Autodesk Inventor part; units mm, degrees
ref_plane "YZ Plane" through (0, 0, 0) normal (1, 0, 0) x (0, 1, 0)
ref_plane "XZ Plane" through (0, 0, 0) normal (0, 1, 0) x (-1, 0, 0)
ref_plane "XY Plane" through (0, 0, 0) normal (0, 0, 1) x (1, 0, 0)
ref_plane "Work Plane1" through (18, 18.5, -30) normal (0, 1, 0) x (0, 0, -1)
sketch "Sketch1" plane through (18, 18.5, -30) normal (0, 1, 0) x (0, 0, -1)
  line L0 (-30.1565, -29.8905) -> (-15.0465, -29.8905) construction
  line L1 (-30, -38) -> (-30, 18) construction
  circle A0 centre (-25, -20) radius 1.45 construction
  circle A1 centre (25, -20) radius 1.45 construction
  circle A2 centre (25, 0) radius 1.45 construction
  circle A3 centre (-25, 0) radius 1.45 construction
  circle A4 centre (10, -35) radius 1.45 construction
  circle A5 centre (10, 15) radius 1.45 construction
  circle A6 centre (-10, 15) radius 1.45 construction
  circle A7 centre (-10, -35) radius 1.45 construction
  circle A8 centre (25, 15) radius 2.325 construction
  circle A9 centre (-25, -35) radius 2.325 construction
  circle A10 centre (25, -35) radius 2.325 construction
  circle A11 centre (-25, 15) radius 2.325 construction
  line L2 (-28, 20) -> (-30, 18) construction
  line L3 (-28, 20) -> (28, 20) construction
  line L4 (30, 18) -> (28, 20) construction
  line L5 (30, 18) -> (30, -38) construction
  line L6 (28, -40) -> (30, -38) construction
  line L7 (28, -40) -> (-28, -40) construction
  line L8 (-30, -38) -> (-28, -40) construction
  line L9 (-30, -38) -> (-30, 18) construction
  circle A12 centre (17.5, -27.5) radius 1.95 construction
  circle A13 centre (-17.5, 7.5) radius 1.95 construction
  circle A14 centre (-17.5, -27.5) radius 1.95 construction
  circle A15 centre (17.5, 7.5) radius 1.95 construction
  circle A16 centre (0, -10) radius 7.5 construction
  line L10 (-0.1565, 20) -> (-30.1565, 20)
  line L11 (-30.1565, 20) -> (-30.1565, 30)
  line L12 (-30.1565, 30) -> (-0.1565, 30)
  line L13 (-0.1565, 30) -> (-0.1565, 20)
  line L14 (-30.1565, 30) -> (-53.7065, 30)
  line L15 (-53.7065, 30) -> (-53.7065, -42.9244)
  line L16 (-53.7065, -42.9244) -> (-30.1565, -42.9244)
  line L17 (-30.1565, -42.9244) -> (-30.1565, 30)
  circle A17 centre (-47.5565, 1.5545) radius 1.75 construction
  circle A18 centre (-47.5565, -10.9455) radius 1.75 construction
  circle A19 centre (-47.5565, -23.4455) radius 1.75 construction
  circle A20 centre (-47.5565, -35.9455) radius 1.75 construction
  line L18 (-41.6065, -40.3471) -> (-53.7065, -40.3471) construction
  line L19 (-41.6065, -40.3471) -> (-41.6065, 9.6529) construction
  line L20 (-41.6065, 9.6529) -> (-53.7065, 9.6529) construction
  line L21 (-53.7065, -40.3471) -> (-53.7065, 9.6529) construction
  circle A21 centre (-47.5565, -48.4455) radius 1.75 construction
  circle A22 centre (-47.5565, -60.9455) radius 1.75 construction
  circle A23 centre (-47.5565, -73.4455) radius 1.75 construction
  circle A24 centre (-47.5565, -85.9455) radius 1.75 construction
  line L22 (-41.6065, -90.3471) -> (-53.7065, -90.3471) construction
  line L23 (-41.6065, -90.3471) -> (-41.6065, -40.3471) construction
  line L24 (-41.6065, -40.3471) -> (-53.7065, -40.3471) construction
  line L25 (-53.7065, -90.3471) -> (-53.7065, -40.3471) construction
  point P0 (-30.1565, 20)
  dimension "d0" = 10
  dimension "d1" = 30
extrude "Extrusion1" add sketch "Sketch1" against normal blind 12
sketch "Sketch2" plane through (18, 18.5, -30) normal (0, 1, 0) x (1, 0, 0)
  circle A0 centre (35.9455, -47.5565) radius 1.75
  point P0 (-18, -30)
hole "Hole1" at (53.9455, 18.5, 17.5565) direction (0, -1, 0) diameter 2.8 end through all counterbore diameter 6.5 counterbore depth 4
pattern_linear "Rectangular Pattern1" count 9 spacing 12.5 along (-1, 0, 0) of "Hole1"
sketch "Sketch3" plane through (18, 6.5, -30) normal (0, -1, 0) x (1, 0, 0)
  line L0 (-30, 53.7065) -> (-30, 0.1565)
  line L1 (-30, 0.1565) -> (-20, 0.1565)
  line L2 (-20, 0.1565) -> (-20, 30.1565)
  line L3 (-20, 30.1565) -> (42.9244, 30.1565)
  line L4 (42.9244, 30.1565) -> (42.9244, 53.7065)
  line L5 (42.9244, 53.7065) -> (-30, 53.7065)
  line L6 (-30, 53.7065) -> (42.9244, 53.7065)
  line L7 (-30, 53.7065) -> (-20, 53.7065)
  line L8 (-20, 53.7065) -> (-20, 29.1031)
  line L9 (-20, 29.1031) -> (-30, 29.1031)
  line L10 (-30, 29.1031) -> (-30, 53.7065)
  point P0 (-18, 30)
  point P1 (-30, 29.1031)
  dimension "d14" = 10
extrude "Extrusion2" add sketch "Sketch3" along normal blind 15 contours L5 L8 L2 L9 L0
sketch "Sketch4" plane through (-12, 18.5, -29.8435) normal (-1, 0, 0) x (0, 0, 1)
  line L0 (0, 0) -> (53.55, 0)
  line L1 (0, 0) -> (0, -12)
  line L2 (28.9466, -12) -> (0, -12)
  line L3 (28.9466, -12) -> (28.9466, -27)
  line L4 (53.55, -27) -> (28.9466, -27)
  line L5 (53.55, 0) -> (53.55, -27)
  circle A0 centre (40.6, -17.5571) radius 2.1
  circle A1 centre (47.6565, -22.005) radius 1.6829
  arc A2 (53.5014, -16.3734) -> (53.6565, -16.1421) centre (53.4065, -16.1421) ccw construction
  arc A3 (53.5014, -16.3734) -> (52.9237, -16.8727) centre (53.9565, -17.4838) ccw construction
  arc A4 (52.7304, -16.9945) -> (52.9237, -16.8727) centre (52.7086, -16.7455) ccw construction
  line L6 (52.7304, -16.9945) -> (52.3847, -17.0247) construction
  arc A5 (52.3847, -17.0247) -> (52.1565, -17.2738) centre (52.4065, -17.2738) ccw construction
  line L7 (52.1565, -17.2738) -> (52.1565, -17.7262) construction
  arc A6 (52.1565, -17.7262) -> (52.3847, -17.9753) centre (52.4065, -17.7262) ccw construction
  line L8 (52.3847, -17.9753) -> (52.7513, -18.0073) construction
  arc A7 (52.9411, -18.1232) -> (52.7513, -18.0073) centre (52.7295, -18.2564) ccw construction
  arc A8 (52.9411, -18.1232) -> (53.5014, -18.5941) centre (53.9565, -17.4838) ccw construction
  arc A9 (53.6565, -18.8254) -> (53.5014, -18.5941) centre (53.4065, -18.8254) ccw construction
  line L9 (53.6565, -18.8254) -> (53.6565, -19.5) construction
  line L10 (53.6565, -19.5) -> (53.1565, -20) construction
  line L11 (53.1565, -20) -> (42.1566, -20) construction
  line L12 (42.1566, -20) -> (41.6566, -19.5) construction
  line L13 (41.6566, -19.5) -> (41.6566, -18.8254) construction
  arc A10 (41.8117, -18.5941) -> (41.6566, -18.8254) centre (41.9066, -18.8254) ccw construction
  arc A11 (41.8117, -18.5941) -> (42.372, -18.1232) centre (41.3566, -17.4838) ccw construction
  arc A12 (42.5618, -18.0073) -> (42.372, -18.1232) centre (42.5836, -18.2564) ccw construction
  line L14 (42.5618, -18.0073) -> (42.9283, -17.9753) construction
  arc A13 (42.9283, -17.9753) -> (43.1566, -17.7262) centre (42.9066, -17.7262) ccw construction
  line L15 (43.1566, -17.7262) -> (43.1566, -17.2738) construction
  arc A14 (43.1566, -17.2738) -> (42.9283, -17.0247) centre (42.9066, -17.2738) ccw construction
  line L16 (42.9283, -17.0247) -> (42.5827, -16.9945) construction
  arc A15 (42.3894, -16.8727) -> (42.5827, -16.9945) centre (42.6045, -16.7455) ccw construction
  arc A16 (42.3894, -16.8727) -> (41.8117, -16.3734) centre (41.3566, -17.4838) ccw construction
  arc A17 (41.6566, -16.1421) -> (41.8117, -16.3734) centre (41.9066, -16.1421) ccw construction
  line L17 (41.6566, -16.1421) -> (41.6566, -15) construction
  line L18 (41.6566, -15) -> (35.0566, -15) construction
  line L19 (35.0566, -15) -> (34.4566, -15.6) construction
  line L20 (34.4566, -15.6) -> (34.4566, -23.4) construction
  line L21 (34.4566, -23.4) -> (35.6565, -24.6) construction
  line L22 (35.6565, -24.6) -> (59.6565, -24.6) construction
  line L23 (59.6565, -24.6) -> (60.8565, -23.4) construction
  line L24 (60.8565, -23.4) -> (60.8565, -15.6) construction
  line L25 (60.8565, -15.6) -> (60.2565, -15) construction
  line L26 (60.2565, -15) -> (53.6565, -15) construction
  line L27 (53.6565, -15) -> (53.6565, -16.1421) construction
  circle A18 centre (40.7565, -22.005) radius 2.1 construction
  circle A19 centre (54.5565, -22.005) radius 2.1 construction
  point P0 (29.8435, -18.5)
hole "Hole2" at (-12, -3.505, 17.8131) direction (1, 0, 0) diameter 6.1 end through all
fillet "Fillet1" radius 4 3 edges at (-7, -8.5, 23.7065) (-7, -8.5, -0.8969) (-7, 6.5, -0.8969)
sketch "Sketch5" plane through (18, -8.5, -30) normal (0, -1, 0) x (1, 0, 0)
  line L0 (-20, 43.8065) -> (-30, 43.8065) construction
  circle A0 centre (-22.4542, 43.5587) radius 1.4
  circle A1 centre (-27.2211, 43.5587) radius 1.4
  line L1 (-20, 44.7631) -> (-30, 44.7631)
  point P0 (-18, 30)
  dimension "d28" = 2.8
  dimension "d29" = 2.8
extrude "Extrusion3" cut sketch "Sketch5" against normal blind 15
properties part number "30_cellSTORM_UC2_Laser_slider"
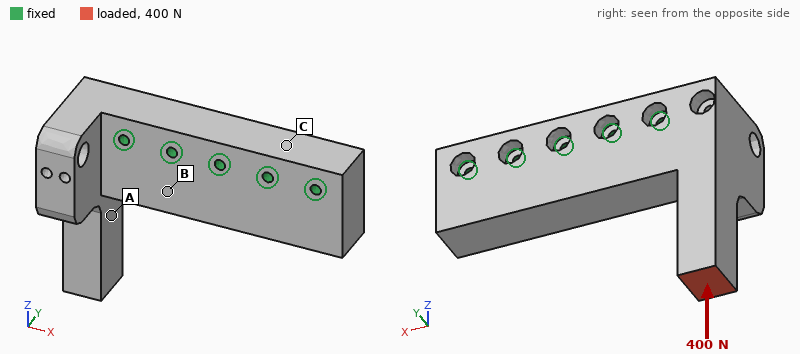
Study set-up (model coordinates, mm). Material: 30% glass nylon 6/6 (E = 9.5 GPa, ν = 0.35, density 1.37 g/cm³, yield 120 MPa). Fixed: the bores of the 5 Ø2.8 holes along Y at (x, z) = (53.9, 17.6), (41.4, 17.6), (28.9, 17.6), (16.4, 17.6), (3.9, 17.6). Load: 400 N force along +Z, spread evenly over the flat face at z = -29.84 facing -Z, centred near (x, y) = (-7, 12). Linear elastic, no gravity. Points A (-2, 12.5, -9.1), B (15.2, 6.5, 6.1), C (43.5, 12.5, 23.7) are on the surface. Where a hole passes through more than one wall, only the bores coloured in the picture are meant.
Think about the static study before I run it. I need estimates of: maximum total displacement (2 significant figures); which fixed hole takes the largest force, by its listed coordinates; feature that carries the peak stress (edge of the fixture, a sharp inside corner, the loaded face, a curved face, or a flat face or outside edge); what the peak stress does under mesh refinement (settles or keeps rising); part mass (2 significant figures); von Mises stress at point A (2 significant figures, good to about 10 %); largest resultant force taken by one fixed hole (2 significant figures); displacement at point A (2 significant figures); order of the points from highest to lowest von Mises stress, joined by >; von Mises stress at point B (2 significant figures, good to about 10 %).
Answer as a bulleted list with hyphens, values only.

- 61 µm
- (3.9, 17.6)
- edge of the fixture
- keeps rising
- 36 g
- 3.3 MPa
- 530 N
- 28 µm
- A > B > C
- 2.4 MPa
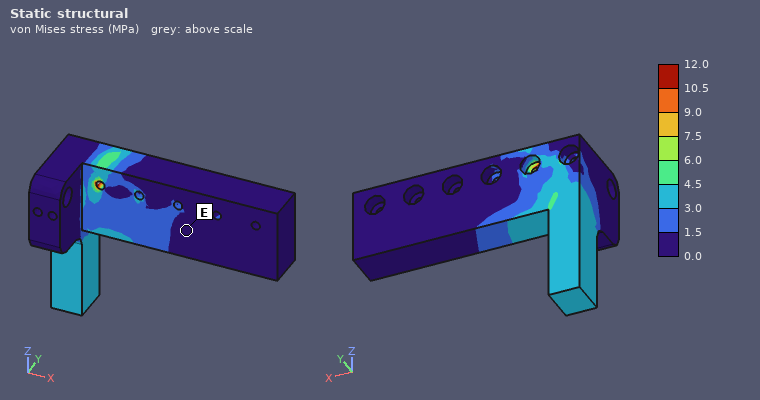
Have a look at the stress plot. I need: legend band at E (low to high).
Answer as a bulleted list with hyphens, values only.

- 0.0 to 1.5 MPa
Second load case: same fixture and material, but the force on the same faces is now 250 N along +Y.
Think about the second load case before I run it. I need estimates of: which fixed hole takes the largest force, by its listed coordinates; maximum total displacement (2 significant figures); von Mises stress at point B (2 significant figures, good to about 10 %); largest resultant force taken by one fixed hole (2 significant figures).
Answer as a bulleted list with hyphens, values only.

- (3.9, 17.6)
- 0.60 mm
- 11 MPa
- 240 N
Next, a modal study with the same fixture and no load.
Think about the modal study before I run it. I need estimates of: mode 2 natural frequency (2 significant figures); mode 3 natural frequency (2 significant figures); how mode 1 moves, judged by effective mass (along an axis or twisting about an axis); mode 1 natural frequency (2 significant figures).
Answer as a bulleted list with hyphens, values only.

- 3000 Hz
- 5100 Hz
- along Y
- 2100 Hz
